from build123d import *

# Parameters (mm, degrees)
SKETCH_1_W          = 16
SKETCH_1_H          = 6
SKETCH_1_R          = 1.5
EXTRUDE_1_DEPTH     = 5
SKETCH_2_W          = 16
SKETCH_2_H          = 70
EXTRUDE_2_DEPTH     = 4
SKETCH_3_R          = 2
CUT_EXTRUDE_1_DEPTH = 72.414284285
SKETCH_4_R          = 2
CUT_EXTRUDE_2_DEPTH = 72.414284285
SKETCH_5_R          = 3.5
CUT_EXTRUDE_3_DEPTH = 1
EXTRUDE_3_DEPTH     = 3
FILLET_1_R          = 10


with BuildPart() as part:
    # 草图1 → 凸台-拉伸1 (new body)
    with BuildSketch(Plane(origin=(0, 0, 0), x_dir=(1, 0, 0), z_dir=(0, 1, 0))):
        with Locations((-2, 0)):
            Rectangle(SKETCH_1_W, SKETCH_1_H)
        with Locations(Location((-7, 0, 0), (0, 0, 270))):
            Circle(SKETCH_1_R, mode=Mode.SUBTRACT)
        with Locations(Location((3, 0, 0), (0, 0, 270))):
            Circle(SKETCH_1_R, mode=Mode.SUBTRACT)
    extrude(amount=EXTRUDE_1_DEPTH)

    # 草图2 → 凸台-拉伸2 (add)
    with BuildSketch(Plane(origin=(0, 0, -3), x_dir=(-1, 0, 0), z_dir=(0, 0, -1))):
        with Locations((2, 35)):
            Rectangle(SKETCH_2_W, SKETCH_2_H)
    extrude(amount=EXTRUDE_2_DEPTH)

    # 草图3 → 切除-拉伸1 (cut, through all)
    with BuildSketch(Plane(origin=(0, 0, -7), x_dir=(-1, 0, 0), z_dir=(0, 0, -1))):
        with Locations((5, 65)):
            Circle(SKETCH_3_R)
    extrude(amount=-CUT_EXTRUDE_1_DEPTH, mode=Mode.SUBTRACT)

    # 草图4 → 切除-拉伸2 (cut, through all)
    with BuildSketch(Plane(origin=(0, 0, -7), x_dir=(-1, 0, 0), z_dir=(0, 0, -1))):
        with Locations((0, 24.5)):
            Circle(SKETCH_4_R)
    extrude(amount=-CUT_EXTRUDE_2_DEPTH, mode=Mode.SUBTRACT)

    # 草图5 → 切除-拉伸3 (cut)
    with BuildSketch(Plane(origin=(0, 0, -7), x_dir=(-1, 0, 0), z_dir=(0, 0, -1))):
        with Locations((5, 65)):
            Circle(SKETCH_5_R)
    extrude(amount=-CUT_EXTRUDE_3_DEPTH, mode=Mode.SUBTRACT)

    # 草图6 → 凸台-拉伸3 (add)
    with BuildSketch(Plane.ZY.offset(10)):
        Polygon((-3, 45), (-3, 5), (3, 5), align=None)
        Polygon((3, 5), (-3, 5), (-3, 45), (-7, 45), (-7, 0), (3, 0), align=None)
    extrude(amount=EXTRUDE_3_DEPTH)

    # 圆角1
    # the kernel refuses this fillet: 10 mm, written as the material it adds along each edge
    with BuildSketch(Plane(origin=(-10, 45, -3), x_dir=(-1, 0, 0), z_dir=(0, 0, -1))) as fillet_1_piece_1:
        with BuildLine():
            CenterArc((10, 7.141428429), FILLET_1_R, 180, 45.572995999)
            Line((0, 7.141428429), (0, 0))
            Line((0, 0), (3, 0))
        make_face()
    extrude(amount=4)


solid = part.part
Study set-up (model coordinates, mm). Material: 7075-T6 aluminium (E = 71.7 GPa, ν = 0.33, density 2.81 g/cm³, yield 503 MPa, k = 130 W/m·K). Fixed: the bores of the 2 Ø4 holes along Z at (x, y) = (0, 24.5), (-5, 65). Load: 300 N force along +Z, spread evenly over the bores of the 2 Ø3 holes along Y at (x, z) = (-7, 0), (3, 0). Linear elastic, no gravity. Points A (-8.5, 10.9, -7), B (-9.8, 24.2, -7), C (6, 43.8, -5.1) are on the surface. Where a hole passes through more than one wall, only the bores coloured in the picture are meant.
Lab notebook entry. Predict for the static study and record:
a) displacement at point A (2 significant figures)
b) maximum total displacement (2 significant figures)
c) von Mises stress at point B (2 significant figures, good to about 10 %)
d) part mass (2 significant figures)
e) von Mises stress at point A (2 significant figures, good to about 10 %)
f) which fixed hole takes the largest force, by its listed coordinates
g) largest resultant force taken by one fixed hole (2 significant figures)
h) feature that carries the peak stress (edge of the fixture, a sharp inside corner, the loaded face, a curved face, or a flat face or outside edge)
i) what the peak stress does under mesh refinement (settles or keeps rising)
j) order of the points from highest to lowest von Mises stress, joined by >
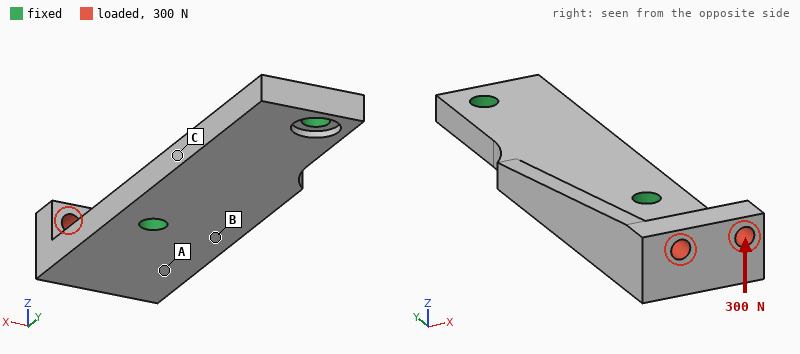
0.058 mm
0.13 mm
50 MPa
16 g
27 MPa
(0, 24.5)
350 N
edge of the fixture
keeps rising
B > A > C
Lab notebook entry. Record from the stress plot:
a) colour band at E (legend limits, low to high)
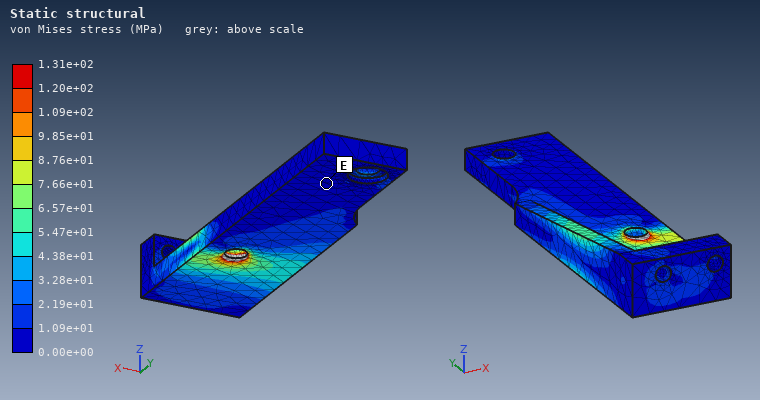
0.00e+00 to 1.09e+01 MPa
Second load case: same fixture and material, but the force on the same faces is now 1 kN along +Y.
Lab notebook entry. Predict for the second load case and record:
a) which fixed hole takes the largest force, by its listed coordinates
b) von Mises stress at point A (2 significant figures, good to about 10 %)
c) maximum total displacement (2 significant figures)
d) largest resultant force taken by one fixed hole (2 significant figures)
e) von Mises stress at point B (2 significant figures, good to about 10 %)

(0, 24.5)
36 MPa
0.14 mm
900 N
44 MPa
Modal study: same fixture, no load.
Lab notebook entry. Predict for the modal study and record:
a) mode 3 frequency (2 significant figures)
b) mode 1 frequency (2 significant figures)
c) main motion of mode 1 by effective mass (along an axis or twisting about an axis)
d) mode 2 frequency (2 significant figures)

11 kHz
4400 Hz
along Z
8200 Hz
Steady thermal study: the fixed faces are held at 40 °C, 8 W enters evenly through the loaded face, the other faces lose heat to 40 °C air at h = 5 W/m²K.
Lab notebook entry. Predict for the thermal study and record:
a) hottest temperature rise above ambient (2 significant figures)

21 K
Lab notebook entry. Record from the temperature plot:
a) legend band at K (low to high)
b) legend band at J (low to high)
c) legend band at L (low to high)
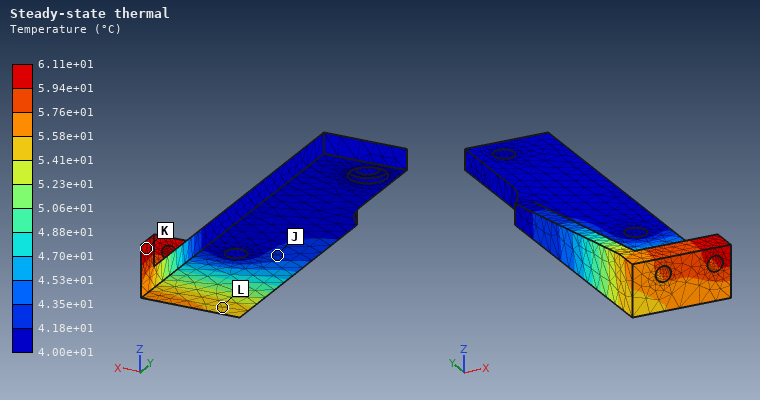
5.94e+01 to 6.11e+01 °C
4.18e+01 to 4.35e+01 °C
5.41e+01 to 5.58e+01 °C
